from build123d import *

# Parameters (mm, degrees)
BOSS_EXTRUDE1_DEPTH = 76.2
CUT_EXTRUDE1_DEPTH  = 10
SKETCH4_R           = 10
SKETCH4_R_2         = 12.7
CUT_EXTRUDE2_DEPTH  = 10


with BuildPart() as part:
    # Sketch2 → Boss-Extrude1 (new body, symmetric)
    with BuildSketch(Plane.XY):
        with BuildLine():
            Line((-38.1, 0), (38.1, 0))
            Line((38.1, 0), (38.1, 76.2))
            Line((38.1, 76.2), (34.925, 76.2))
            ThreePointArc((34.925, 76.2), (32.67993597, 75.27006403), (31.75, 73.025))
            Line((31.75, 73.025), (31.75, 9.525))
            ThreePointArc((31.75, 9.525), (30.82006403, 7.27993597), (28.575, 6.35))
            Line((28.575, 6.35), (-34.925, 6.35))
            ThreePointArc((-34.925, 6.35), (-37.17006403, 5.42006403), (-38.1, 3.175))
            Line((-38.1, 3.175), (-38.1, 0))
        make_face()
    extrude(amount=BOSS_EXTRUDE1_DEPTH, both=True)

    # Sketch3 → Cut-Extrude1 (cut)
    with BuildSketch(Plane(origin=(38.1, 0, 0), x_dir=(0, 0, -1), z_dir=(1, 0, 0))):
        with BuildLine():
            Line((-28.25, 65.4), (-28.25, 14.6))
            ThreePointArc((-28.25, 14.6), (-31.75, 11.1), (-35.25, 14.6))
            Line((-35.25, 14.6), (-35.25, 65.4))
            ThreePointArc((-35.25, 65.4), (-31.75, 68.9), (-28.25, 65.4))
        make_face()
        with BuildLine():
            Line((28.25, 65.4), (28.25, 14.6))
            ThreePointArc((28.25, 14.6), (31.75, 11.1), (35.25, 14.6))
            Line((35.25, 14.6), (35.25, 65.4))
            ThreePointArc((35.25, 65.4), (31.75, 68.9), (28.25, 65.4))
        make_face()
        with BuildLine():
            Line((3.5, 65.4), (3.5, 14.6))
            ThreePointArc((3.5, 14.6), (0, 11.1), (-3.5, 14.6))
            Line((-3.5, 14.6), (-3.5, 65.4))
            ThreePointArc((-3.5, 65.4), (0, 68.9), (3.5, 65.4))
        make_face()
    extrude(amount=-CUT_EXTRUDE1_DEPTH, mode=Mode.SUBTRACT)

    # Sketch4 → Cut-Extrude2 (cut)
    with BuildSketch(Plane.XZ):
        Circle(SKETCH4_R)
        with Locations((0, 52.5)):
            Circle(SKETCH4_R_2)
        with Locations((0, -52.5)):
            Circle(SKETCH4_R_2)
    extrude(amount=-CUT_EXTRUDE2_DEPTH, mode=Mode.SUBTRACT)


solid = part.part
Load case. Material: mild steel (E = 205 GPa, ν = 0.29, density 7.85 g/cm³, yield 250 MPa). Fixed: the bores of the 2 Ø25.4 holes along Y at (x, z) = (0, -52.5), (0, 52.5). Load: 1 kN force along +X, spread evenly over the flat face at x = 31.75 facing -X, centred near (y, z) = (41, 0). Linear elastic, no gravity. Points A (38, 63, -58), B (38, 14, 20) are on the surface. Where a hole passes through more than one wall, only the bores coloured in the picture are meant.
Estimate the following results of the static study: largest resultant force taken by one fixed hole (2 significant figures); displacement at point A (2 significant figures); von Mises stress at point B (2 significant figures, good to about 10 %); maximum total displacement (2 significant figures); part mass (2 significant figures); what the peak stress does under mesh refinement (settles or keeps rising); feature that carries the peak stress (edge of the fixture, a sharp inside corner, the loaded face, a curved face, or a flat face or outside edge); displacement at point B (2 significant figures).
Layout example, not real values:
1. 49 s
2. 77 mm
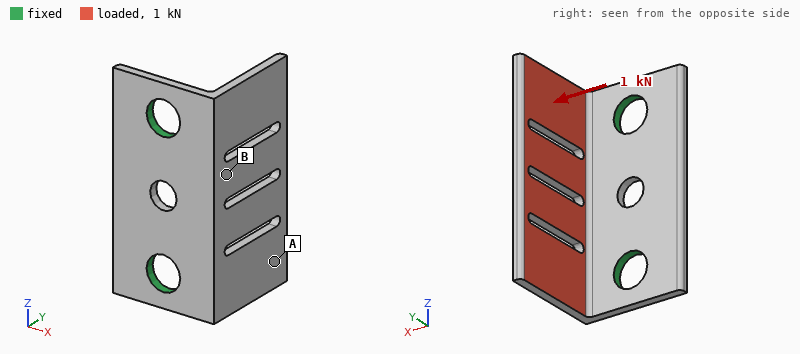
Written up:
1. 500 N
2. 0.14 mm
3. 28 MPa
4. 0.18 mm
5. 980 g
6. keeps rising
7. edge of the fixture
8. 0.031 mm
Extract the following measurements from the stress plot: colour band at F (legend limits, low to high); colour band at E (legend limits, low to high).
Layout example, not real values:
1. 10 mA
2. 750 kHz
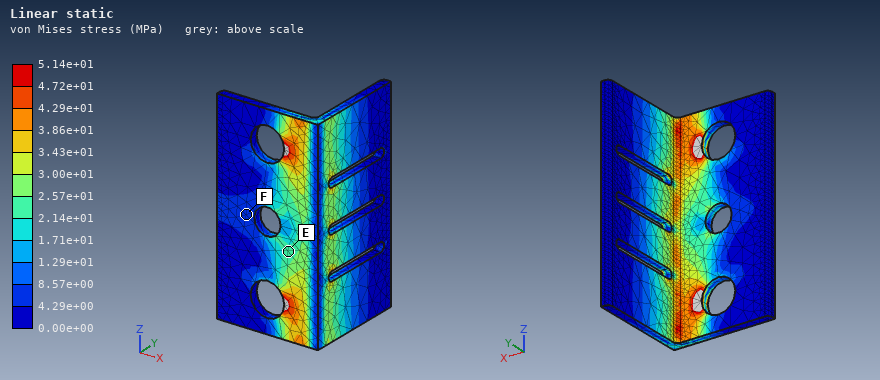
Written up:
1. 4.29e+00 to 8.57e+00 MPa
2. 2.14e+01 to 2.57e+01 MPa
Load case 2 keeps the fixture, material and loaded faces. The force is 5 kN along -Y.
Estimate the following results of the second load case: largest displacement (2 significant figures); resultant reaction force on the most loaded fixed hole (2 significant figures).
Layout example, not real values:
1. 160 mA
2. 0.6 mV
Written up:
1. 0.13 mm
2. 2.5 kN
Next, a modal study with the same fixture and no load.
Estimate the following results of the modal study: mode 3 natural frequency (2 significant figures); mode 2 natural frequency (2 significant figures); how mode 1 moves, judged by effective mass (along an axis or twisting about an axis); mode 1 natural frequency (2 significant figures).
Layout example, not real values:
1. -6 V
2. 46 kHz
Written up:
1. 2300 Hz
2. 1100 Hz
3. along X
4. 670 Hz
